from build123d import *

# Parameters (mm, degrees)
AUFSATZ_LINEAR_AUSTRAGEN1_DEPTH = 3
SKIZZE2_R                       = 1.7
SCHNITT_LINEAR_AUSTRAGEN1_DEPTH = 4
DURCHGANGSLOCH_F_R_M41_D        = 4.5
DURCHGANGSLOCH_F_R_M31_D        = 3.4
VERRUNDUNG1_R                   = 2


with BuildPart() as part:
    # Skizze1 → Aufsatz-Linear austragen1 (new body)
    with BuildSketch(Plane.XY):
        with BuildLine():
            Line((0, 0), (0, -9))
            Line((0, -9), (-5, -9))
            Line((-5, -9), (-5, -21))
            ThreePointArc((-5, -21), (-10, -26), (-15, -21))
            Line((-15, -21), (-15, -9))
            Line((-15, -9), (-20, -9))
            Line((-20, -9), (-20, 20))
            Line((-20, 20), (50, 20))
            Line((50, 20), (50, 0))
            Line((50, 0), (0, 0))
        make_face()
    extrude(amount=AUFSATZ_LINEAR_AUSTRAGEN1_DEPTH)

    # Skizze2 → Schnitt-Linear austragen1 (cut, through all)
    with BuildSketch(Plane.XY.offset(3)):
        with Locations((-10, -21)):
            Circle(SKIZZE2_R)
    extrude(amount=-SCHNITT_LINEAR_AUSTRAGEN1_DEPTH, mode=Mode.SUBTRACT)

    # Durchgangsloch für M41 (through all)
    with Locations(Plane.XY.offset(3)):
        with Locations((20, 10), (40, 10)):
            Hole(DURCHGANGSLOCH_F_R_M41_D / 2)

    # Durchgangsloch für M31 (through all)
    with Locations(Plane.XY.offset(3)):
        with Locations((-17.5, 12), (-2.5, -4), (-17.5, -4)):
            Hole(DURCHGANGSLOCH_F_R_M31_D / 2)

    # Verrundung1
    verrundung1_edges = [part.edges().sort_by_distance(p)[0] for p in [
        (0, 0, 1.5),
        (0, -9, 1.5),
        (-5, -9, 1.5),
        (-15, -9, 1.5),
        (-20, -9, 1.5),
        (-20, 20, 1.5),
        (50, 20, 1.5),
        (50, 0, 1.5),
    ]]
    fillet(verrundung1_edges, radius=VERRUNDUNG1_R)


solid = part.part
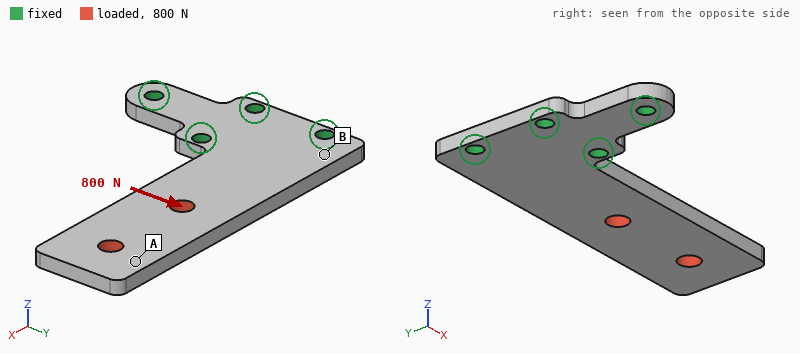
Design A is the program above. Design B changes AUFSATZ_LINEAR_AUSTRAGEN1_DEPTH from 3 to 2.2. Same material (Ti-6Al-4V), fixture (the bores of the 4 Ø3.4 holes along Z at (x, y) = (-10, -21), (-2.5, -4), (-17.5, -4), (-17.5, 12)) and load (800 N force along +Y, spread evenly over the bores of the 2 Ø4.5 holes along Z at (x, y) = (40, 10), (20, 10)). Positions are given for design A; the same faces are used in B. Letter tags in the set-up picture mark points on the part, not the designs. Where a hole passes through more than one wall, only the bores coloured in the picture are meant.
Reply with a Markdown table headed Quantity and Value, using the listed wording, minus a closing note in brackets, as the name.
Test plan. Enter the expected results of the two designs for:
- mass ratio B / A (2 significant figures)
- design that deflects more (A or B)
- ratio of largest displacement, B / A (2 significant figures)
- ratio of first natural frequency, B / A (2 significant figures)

| Quantity | Value |
|---|---|
| mass ratio B / A | 0.73 |
| design that deflects more | B |
| ratio of largest displacement, B / A | 1.4 |
| ratio of first natural frequency, B / A | 0.74 |
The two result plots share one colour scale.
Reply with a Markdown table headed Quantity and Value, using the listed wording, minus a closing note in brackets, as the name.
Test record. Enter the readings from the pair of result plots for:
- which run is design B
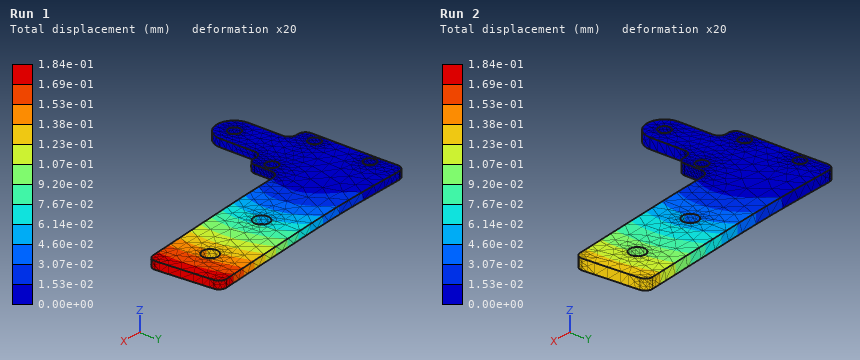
| Quantity | Value |
|---|---|
| which run is design B | Run 1 |
